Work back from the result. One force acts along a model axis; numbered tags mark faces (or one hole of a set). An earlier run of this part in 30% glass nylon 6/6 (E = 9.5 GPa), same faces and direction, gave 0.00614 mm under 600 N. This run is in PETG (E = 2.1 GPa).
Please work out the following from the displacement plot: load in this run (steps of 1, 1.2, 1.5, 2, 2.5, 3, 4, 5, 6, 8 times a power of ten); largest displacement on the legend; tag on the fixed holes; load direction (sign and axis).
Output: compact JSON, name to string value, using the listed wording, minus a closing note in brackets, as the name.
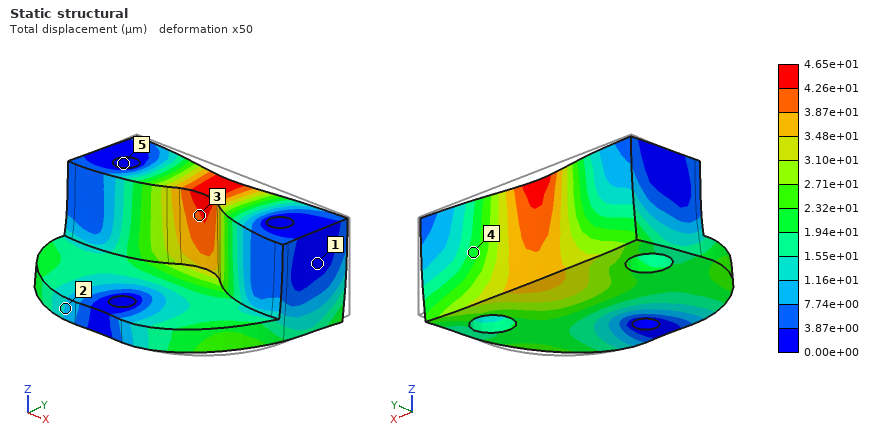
{"load in this run": "1 kN", "largest displacement on the legend": "4.65e+01 µm", "tag on the fixed holes": "5", "load direction": "-Y"}
